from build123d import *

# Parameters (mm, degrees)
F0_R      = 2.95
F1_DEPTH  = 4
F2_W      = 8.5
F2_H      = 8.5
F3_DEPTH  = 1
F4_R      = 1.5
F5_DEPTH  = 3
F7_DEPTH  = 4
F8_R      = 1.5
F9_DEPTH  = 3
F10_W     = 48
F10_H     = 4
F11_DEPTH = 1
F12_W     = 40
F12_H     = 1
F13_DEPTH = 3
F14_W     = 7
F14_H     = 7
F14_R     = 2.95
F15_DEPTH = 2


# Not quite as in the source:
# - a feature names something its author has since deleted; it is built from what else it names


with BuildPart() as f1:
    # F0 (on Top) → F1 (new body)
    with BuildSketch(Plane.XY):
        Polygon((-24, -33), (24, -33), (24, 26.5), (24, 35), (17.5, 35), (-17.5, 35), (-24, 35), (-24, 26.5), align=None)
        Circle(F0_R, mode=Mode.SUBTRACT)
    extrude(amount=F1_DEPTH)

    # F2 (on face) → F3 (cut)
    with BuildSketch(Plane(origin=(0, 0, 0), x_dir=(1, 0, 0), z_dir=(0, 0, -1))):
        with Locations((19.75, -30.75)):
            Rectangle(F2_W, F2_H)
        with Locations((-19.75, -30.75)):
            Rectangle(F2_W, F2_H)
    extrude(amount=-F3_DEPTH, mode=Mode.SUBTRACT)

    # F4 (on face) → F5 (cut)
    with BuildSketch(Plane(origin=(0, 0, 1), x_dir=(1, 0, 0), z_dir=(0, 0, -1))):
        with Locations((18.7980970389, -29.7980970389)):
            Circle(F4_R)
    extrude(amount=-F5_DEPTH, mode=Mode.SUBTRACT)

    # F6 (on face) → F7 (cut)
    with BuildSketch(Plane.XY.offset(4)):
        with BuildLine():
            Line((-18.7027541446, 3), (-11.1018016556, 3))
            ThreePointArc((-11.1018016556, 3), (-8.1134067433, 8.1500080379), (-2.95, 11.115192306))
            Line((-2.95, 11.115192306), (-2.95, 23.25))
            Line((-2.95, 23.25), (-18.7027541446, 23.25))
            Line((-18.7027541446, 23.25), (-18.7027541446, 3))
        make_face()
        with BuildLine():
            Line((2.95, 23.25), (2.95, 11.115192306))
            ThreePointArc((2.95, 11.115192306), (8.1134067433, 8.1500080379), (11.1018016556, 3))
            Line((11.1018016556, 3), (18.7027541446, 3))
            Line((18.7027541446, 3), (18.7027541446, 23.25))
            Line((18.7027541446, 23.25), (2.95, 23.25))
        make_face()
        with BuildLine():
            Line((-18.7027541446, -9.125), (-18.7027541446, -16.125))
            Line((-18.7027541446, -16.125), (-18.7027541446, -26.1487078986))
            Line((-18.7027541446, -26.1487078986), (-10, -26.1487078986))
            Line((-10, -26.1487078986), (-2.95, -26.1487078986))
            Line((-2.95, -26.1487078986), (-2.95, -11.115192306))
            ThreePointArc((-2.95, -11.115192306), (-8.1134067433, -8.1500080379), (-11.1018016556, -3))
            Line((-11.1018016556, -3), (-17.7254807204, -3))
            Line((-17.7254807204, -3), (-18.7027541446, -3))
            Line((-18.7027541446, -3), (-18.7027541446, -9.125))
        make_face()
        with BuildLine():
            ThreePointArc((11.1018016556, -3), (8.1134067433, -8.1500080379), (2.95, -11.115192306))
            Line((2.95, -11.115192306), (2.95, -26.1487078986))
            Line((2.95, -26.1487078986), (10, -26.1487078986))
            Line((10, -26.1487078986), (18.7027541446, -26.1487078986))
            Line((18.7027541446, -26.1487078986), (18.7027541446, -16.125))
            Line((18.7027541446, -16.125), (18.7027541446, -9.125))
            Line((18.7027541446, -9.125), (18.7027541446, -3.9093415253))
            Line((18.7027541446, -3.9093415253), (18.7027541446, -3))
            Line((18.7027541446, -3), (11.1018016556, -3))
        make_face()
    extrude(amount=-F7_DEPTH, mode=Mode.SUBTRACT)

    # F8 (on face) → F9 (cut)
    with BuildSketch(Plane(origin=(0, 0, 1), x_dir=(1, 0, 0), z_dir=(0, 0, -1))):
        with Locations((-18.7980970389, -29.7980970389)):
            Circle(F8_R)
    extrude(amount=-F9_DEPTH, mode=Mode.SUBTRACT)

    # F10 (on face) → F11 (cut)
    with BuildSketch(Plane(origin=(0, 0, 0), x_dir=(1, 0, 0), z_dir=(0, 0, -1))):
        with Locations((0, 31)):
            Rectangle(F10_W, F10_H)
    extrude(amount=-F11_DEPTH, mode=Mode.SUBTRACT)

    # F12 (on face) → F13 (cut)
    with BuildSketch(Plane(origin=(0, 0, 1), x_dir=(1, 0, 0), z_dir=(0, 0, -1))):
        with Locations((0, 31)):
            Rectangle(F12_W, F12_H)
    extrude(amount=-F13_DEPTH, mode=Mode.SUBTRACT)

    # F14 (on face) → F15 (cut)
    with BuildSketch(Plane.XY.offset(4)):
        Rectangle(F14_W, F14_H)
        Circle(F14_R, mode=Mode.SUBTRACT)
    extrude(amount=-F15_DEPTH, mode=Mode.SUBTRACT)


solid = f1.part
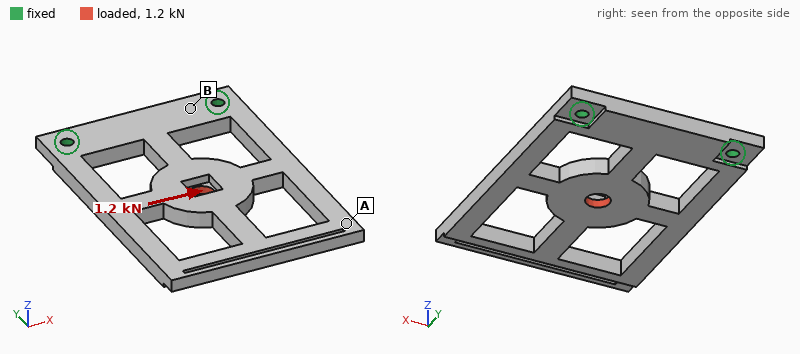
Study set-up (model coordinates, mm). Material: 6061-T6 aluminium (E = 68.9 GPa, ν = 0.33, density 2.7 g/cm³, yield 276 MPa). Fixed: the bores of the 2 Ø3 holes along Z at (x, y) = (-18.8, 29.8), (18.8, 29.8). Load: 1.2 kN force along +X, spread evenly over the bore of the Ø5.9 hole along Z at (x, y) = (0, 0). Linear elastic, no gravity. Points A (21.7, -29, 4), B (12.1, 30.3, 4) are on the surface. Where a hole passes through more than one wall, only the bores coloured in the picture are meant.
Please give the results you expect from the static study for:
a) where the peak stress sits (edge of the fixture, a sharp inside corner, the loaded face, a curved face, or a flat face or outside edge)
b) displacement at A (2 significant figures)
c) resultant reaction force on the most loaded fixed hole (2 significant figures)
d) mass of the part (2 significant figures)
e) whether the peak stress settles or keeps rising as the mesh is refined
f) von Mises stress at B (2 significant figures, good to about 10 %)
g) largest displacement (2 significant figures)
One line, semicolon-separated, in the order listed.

a sharp inside corner; 0.14 mm; 1.1 kN; 21 g; keeps rising; 30 MPa; 0.15 mm
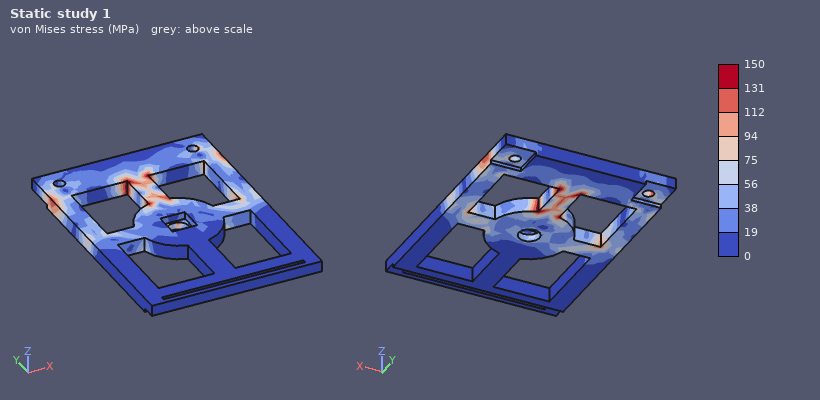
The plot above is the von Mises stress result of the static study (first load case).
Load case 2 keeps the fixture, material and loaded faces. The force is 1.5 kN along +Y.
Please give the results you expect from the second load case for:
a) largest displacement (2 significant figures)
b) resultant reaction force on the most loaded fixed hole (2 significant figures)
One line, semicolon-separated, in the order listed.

0.37 mm; 760 N
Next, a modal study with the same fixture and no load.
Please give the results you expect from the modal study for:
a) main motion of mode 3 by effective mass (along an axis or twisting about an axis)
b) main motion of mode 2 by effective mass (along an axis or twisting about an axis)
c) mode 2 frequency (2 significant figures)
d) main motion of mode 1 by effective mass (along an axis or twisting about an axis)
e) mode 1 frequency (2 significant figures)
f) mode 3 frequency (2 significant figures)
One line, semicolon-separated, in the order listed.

along X; twisting about Y; 1800 Hz; along Z; 650 Hz; 3700 Hz
